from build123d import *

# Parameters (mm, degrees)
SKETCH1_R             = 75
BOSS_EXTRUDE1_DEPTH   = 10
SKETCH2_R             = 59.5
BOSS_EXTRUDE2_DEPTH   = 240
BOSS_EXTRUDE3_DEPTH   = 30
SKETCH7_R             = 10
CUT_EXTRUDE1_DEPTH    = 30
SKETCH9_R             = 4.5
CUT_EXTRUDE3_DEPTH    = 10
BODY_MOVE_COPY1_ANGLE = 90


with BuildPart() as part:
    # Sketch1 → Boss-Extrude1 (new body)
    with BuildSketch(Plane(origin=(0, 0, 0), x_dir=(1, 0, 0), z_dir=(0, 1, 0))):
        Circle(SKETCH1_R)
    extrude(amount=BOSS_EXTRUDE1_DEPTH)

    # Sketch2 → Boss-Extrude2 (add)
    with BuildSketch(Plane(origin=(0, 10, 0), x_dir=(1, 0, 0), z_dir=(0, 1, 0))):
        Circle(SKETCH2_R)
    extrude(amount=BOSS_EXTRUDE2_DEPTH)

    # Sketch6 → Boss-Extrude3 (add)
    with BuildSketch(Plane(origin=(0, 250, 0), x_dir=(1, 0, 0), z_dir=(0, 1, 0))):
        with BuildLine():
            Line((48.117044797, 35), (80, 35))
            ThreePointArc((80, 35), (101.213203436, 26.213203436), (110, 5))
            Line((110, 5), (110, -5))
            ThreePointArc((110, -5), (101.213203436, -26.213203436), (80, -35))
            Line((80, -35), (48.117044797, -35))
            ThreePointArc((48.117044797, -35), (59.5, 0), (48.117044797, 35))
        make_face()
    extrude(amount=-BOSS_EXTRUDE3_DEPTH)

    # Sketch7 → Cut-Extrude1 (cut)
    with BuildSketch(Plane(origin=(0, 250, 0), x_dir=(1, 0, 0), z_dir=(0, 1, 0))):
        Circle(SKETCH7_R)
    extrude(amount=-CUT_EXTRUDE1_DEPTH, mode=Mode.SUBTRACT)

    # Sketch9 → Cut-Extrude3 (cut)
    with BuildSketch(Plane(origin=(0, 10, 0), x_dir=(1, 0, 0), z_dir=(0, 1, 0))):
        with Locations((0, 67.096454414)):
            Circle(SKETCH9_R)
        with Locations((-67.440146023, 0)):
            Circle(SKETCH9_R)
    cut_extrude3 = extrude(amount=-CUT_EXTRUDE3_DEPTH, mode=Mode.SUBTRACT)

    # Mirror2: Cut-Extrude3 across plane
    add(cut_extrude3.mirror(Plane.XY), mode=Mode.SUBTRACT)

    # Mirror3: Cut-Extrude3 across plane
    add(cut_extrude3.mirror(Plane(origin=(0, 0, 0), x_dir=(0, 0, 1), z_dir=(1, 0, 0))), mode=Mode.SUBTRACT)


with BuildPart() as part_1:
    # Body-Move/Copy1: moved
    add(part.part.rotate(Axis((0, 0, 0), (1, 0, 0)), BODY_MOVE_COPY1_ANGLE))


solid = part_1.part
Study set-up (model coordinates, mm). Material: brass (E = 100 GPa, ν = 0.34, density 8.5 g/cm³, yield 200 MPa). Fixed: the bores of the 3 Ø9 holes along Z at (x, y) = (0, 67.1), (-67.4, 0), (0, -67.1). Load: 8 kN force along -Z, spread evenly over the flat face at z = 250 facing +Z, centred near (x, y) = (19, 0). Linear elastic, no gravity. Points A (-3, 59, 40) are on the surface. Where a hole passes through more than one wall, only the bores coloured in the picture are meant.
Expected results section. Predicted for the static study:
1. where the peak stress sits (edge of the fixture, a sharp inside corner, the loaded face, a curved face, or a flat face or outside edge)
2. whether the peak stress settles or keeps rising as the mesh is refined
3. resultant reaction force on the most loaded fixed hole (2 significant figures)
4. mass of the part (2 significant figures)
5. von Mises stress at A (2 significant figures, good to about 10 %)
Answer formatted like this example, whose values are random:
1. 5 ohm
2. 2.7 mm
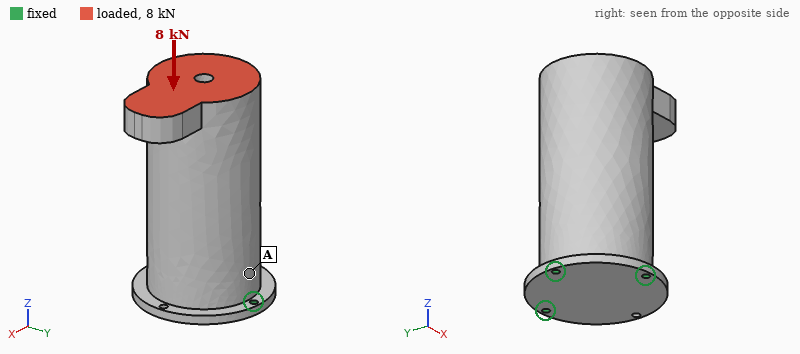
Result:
1. edge of the fixture
2. keeps rising
3. 5.5 kN
4. 25 kg
5. 4.1 MPa
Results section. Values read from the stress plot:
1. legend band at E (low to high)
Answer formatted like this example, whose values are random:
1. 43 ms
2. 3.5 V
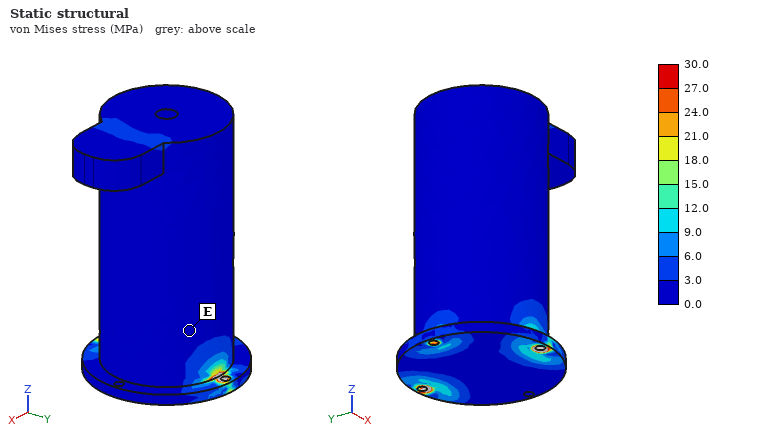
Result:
1. 0.0 to 3.0 MPa
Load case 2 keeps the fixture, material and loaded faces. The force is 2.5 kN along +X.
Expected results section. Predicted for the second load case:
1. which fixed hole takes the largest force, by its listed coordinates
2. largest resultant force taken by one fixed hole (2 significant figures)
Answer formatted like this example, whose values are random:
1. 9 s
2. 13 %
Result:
1. (-67.4, 0)
2. 9.8 kN
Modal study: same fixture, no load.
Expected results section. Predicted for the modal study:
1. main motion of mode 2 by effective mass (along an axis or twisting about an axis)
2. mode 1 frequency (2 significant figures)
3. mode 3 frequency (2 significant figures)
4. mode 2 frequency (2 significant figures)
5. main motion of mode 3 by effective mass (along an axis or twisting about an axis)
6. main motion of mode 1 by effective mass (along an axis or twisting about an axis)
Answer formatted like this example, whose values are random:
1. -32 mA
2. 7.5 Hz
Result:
1. along Y
2. 240 Hz
3. 1200 Hz
4. 400 Hz
5. along Z
6. along X
